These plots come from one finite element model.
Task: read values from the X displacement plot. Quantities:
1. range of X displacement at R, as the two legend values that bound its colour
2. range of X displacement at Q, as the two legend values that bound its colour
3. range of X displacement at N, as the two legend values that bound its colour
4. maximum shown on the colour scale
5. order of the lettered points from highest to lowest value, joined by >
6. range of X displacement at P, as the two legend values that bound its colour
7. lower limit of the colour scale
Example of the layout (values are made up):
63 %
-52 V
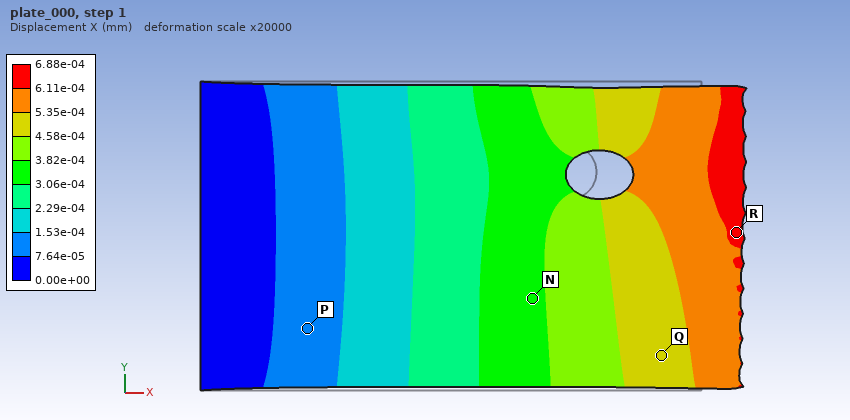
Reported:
6.11e-04 to 6.88e-04 mm
4.58e-04 to 5.35e-04 mm
3.06e-04 to 3.82e-04 mm
6.88e-04 mm
R > Q > N > P
7.64e-05 to 1.53e-04 mm
0.00e+00 mm
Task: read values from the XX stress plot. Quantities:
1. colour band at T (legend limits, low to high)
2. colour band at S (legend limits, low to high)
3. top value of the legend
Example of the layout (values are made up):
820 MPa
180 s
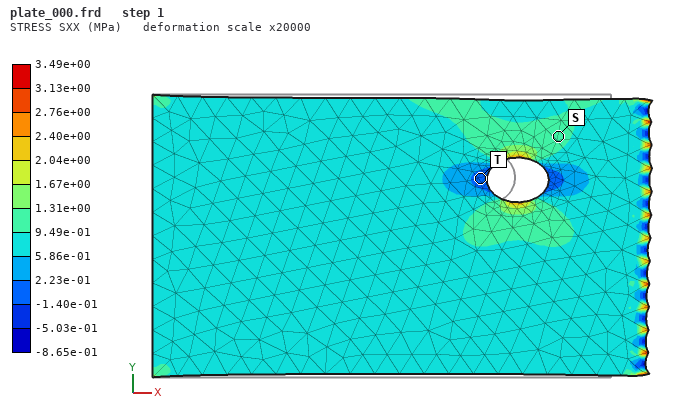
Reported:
-1.40e-01 to 2.23e-01 MPa
9.49e-01 to 1.31e+00 MPa
3.49e+00 MPa
